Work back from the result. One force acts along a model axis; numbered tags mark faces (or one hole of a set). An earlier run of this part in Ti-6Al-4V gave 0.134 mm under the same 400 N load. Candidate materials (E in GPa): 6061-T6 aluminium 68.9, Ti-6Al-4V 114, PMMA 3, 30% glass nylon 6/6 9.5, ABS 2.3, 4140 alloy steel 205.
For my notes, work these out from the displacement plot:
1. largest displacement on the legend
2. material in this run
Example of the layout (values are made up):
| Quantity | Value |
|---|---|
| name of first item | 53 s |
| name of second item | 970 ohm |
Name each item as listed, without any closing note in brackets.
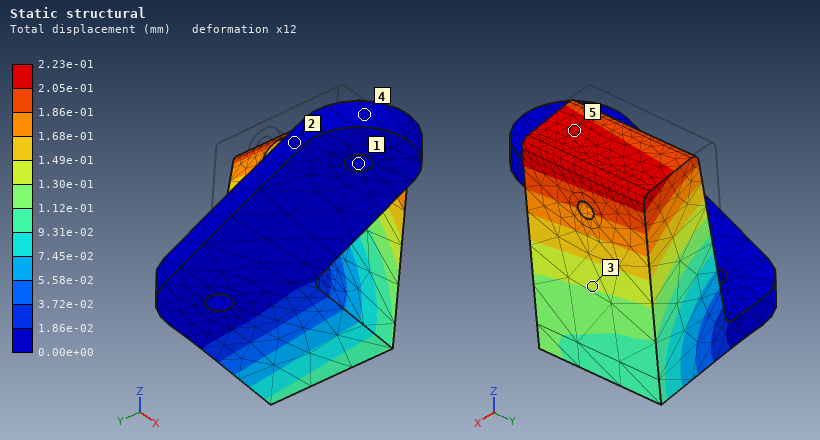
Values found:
| Quantity | Value |
|---|---|
| largest displacement on the legend | 2.23e-01 mm |
| material in this run | 6061-T6 aluminium |
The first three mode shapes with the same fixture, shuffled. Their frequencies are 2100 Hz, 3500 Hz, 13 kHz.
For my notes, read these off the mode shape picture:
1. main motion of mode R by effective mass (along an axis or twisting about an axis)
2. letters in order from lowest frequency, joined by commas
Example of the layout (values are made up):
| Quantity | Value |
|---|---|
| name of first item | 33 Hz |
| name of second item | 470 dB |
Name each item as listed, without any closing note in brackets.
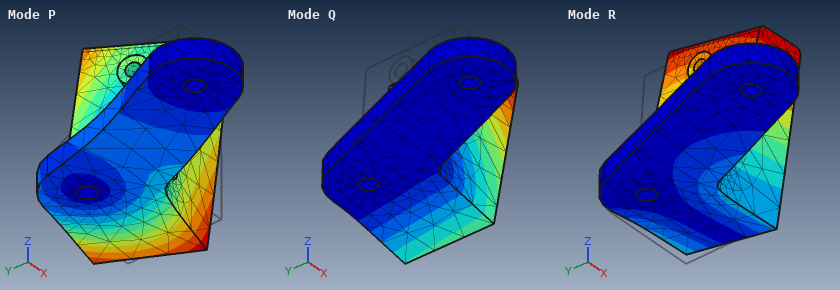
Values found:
| Quantity | Value |
|---|---|
| main motion of mode R by effective mass | along Y |
| letters in order from lowest frequency, joined by commas | Q, R, P |
